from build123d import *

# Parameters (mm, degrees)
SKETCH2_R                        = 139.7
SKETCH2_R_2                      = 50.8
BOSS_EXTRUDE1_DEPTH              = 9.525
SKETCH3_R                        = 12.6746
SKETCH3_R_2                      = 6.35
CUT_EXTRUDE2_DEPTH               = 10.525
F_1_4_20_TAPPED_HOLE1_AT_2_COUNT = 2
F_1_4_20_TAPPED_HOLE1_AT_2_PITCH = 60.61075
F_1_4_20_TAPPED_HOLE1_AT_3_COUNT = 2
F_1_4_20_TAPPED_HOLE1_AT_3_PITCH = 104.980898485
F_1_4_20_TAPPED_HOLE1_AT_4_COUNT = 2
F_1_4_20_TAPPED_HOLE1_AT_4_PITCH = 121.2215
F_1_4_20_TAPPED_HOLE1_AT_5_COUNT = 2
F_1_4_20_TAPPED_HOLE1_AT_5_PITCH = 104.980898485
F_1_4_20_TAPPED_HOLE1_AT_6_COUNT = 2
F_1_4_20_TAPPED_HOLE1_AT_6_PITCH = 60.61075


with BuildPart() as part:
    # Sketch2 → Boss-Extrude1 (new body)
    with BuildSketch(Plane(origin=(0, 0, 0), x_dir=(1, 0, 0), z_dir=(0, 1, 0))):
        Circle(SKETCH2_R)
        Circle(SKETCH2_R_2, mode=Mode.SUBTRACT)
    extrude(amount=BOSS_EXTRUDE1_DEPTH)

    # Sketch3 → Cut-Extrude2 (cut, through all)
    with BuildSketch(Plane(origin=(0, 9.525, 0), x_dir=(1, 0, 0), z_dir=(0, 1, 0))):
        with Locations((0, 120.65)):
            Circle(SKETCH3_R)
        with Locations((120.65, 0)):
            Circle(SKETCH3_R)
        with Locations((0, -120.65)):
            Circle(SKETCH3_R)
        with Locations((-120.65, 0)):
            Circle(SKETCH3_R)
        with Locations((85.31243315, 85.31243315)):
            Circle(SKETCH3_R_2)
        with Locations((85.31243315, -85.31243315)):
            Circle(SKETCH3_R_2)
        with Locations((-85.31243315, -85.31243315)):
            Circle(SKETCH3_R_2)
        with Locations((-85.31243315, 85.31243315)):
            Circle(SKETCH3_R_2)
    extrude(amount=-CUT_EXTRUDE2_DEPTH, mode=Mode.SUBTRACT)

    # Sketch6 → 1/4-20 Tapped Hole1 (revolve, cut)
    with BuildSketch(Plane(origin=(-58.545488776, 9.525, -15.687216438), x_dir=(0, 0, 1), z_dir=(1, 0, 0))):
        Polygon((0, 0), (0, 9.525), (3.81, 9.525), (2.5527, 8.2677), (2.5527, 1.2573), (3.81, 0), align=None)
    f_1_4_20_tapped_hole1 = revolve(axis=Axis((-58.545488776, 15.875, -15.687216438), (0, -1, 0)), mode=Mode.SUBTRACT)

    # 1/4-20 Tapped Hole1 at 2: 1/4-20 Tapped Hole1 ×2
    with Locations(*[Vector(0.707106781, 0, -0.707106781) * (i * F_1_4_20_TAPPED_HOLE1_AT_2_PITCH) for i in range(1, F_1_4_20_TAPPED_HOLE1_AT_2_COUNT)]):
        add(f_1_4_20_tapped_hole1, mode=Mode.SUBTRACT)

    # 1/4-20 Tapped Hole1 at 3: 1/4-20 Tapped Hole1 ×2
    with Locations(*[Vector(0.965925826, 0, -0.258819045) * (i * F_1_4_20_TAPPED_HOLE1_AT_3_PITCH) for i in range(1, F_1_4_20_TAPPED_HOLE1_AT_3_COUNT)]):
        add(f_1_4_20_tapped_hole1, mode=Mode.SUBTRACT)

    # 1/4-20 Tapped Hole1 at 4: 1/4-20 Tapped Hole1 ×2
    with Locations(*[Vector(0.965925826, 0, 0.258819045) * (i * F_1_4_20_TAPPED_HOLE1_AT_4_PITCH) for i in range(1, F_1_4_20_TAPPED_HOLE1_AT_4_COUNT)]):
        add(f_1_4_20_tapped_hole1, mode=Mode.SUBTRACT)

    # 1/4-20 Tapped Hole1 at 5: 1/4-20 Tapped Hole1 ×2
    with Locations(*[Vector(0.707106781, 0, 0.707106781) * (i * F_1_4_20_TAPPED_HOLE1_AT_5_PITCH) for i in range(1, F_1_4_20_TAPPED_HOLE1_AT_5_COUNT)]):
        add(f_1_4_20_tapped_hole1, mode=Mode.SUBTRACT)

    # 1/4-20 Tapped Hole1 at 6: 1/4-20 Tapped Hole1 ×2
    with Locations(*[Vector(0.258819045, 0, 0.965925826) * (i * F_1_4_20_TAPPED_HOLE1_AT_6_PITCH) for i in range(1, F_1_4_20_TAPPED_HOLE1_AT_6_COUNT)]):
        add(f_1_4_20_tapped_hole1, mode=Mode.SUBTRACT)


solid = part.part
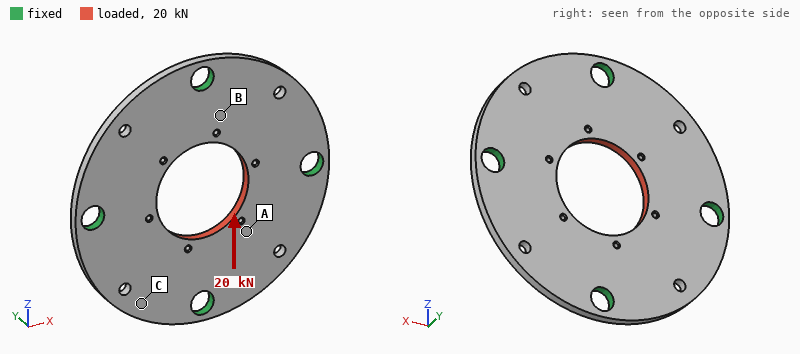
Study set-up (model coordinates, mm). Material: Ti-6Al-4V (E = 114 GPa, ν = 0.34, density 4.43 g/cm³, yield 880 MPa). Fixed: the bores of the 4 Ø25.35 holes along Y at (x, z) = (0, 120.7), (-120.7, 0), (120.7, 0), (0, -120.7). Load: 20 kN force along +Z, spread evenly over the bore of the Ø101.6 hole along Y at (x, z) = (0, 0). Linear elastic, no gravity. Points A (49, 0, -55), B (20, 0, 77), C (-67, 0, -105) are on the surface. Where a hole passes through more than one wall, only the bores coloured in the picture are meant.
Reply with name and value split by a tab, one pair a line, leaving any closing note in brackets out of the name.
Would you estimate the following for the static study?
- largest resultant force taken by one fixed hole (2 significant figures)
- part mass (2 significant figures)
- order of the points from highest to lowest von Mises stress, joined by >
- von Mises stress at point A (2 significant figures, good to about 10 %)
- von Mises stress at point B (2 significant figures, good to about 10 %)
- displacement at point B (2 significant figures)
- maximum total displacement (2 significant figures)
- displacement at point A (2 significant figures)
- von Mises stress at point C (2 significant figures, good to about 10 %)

largest resultant force taken by one fixed hole	6.1 kN
part mass	2.1 kg
order of the points from highest to lowest von Mises stress, joined by >	B > A > C
von Mises stress at point A	5.8 MPa
von Mises stress at point B	9.5 MPa
displacement at point B	4.0 µm
maximum total displacement	8.1 µm
displacement at point A	5.9 µm
von Mises stress at point C	2.5 MPa
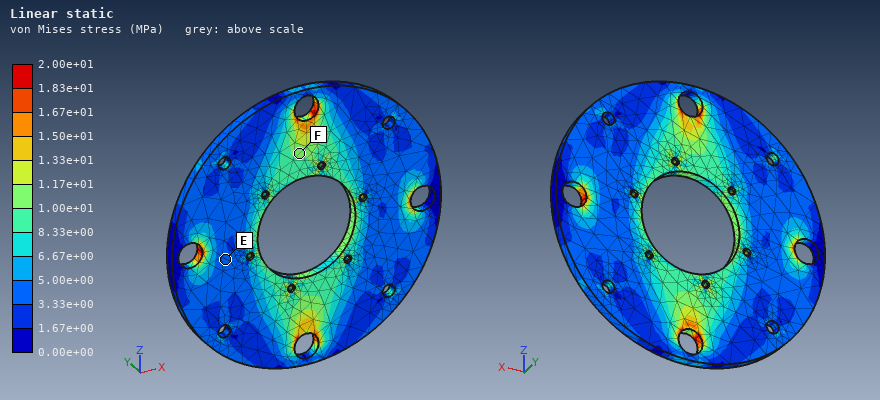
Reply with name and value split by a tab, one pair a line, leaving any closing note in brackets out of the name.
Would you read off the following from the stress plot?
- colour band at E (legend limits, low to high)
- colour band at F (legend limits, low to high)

colour band at E	3.33e+00 to 5.00e+00 MPa
colour band at F	1.00e+01 to 1.17e+01 MPa
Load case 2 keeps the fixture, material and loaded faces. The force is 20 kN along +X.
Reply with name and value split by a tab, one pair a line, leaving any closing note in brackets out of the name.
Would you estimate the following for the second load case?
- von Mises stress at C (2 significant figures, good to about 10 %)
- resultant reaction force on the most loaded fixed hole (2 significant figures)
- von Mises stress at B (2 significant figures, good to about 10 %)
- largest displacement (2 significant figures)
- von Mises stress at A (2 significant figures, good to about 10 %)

von Mises stress at C	3.1 MPa
resultant reaction force on the most loaded fixed hole	6.1 kN
von Mises stress at B	3.8 MPa
largest displacement	8.1 µm
von Mises stress at A	5.8 MPa
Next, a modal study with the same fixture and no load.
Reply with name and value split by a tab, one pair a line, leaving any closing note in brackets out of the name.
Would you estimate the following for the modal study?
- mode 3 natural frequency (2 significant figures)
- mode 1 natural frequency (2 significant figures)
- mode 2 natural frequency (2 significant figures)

mode 3 natural frequency	1800 Hz
mode 1 natural frequency	1700 Hz
mode 2 natural frequency	1800 Hz
